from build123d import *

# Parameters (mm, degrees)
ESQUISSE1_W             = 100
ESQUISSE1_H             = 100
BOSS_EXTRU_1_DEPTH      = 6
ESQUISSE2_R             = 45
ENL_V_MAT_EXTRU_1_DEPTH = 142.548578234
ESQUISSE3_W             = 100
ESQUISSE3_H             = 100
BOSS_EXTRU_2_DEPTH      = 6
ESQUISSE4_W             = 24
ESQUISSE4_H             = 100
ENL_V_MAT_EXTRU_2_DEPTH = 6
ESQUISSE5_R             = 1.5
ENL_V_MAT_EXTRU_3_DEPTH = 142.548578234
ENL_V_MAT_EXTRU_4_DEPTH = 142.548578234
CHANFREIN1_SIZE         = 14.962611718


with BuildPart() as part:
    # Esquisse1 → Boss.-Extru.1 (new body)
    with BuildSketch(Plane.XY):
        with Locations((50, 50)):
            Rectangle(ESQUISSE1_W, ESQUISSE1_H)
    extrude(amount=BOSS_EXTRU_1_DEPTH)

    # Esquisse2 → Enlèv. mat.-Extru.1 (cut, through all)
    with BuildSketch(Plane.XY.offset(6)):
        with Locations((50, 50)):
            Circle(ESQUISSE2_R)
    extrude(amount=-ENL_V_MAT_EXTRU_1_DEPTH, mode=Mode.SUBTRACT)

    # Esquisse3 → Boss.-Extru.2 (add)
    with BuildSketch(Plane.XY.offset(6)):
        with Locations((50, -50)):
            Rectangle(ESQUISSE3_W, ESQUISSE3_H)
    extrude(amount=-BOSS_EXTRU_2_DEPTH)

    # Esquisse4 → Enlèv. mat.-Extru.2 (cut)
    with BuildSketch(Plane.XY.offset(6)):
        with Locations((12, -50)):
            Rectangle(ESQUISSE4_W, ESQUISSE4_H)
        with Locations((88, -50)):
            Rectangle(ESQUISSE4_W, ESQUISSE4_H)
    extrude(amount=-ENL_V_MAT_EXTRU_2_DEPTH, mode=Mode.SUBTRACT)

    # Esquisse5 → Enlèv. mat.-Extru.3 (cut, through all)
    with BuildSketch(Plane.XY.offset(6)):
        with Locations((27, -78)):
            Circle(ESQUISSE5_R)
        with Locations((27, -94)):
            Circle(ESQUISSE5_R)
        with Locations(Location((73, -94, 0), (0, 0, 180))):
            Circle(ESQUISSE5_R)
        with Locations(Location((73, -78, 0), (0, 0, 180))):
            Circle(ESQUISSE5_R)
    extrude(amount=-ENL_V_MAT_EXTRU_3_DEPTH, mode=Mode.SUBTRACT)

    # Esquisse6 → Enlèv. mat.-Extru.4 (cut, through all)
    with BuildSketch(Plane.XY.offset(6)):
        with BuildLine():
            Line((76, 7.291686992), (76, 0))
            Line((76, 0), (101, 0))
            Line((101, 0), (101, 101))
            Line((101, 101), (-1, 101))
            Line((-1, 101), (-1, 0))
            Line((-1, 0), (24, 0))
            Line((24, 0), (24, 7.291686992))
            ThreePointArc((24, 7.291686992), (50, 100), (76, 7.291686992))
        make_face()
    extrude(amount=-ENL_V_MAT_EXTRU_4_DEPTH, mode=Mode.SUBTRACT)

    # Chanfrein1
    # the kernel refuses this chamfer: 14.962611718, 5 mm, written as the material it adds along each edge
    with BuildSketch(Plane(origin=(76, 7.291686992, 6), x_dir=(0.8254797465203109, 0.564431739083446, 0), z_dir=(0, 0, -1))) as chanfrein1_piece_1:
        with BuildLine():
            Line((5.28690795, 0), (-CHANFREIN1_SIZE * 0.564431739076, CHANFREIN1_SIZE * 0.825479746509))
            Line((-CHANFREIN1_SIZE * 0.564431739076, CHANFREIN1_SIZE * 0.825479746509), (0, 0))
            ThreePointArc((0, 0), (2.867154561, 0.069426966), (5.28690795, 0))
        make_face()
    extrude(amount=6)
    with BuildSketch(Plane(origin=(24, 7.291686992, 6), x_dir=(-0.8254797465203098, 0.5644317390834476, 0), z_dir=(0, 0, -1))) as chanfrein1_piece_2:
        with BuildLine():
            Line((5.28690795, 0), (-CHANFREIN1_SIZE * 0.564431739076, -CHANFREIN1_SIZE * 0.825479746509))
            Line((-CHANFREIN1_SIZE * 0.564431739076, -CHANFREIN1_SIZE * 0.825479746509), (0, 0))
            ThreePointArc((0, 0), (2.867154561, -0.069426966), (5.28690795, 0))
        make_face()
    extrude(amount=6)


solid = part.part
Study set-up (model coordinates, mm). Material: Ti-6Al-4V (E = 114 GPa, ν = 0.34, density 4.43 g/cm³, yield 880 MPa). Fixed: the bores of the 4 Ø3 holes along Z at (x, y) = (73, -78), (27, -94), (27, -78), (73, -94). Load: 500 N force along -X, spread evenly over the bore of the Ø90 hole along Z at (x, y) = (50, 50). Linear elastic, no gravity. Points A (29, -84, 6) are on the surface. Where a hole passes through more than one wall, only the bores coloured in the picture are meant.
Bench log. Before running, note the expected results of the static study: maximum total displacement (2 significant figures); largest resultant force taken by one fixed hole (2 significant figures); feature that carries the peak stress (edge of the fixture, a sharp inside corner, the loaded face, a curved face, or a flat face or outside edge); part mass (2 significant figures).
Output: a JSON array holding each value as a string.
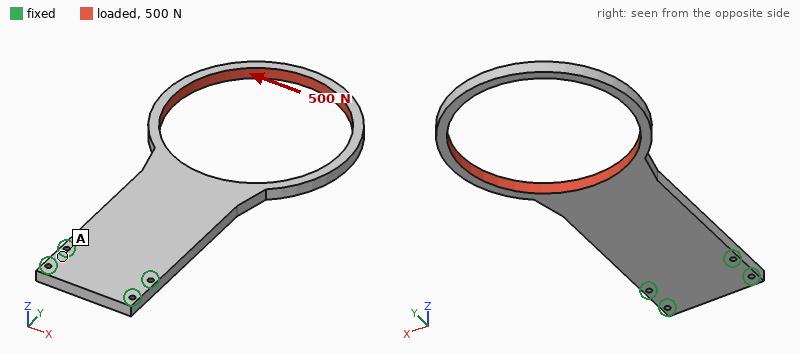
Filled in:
["1.3 mm", "1.3 kN", "the loaded face", "180 g"]
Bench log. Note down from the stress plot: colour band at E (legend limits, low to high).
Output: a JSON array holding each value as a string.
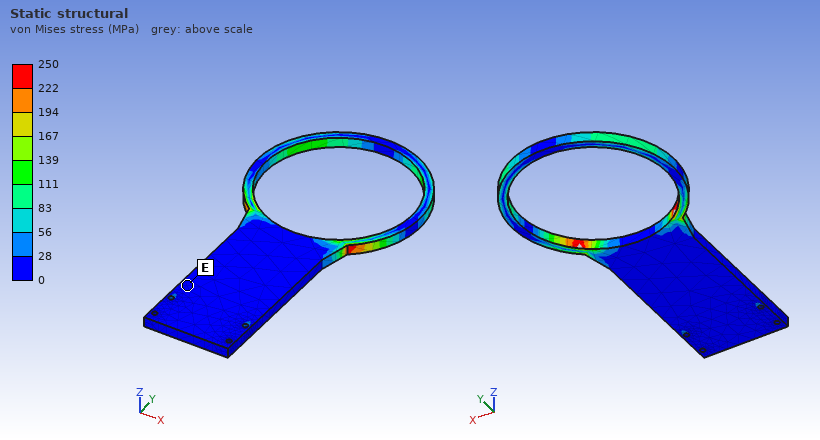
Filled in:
["0 to 28 MPa"]
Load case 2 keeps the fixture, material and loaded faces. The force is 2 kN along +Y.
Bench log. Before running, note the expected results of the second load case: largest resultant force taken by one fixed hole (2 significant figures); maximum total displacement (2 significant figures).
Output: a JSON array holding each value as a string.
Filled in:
["770 N", "0.66 mm"]
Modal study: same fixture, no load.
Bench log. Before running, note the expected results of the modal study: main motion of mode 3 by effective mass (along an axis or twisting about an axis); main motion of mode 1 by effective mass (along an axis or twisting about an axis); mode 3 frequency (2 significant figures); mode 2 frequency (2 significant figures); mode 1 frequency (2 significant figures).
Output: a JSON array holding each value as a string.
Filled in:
["twisting about Y", "along Z", "640 Hz", "530 Hz", "220 Hz"]
